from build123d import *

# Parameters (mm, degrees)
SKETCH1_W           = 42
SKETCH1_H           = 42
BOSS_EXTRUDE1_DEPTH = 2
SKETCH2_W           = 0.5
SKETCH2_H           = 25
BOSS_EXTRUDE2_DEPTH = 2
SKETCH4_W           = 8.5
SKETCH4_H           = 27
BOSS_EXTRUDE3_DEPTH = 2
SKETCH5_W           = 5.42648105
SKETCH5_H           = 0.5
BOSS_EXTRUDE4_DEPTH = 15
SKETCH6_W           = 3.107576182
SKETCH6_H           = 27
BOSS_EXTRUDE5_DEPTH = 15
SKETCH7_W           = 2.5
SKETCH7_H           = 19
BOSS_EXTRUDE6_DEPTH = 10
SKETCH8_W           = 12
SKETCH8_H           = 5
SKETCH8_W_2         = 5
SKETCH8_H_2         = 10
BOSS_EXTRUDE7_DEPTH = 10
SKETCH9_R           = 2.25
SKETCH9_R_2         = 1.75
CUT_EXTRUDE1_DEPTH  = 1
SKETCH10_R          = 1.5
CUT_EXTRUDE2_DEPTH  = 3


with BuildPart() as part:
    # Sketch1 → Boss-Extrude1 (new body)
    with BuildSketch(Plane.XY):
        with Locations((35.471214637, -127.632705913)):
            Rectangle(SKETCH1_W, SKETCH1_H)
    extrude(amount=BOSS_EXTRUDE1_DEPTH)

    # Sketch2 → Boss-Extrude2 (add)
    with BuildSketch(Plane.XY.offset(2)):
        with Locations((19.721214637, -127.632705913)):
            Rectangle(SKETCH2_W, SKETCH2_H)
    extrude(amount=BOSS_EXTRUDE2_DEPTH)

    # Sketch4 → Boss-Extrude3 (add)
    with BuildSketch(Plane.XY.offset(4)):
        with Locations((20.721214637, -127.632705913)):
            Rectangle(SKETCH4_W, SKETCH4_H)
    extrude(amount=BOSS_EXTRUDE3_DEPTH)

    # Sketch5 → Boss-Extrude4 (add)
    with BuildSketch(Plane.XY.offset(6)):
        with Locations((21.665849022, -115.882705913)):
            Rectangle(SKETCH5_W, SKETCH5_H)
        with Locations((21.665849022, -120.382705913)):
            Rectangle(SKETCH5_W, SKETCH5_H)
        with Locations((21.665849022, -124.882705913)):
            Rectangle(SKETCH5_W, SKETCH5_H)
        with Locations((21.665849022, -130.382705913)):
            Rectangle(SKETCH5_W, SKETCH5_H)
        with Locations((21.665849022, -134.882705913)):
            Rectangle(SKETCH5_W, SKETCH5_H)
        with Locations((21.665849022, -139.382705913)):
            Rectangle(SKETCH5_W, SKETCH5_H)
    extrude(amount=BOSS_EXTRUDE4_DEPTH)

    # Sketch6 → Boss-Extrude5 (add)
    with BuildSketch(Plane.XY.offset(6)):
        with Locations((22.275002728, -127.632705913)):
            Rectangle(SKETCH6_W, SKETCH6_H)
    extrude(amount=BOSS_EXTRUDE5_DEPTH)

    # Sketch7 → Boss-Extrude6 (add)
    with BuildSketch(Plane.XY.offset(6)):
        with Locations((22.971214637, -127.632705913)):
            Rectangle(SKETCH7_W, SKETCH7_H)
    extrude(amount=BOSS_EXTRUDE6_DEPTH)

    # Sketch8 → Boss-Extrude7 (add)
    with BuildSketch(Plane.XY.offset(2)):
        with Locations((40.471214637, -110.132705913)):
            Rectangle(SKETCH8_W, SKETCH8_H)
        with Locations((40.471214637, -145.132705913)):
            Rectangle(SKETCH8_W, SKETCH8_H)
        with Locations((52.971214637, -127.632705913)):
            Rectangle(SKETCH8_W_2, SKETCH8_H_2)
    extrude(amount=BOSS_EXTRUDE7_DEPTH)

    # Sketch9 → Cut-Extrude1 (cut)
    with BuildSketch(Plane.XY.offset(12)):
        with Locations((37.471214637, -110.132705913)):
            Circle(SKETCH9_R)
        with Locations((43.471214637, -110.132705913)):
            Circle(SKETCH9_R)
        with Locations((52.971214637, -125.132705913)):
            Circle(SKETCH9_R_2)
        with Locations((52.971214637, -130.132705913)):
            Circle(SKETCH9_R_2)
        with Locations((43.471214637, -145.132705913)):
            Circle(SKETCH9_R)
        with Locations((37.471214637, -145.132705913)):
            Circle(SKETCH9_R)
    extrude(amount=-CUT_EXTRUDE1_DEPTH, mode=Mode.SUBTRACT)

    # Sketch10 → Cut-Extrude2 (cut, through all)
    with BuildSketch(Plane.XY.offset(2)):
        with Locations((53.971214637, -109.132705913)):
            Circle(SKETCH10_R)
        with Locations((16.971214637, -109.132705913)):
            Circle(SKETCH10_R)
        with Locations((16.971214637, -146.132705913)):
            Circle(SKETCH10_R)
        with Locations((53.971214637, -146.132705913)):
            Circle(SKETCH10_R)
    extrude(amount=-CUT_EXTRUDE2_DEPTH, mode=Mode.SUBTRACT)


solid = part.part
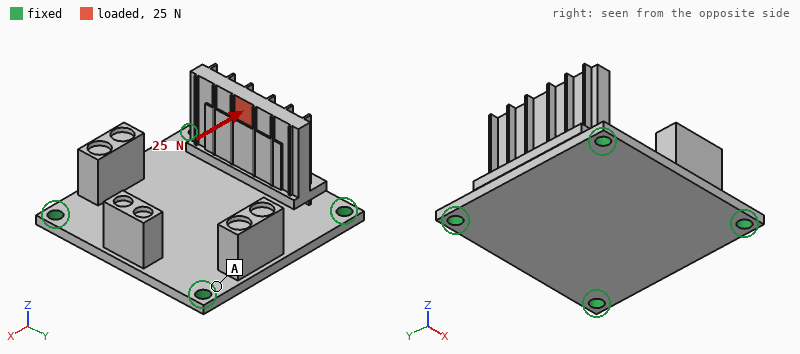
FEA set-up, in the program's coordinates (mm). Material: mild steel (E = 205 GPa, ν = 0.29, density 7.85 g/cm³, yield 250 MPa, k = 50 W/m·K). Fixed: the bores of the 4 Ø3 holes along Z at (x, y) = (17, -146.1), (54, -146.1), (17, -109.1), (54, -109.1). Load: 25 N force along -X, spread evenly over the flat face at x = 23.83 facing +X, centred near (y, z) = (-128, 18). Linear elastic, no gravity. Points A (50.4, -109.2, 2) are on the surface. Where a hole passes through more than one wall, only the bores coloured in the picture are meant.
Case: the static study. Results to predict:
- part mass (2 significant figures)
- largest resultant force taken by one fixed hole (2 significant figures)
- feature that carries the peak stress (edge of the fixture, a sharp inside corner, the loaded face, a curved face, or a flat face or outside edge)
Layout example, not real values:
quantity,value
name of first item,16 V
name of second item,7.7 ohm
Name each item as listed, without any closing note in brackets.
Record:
quantity,value
part mass,55 g
largest resultant force taken by one fixed hole,9.3 N
feature that carries the peak stress,a flat face or outside edge
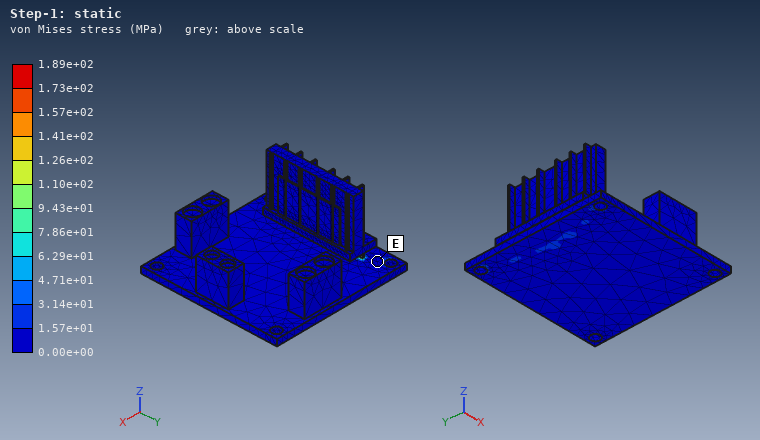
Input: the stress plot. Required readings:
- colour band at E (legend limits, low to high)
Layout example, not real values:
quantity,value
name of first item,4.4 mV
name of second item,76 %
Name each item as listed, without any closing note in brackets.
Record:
quantity,value
colour band at E,0.00e+00 to 1.57e+01 MPa
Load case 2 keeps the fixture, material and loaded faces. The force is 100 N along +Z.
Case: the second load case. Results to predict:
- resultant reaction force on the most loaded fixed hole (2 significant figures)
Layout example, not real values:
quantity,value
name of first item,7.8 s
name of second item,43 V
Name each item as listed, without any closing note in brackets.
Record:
quantity,value
resultant reaction force on the most loaded fixed hole,46 N
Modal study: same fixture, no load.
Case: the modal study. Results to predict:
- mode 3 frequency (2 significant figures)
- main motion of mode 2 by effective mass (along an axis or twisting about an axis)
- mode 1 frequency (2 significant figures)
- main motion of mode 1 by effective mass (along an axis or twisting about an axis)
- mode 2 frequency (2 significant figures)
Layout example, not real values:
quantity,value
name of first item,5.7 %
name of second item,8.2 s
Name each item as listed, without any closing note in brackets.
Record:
quantity,value
mode 3 frequency,6200 Hz
main motion of mode 2 by effective mass,along Z
mode 1 frequency,640 Hz
main motion of mode 1 by effective mass,along X
mode 2 frequency,4800 Hz
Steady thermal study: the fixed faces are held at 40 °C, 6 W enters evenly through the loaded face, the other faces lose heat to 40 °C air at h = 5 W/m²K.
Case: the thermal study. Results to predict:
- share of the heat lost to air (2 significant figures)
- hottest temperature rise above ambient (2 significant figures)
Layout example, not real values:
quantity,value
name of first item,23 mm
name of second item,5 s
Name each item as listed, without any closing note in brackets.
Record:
quantity,value
share of the heat lost to air,11 %
hottest temperature rise above ambient,74 K
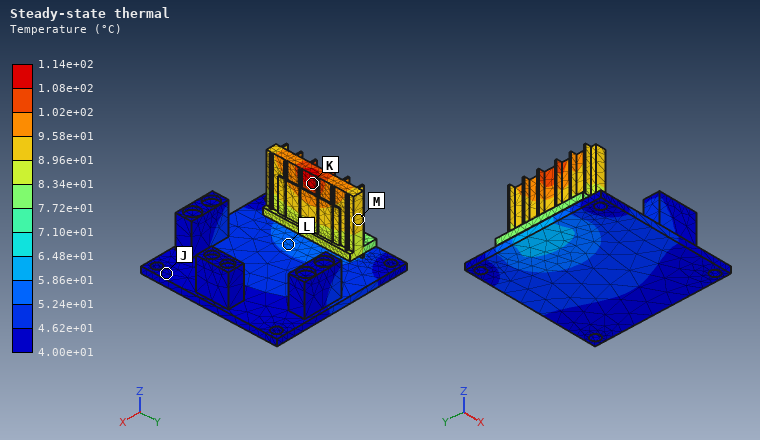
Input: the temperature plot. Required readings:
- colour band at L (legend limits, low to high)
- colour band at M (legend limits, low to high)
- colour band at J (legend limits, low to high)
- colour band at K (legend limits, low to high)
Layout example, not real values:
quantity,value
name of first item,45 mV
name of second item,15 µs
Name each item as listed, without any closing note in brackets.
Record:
quantity,value
colour band at L,5.24e+01 to 5.86e+01 °C
colour band at M,8.96e+01 to 9.58e+01 °C
colour band at J,4.00e+01 to 4.62e+01 °C
colour band at K,1.08e+02 to 1.14e+02 °C
